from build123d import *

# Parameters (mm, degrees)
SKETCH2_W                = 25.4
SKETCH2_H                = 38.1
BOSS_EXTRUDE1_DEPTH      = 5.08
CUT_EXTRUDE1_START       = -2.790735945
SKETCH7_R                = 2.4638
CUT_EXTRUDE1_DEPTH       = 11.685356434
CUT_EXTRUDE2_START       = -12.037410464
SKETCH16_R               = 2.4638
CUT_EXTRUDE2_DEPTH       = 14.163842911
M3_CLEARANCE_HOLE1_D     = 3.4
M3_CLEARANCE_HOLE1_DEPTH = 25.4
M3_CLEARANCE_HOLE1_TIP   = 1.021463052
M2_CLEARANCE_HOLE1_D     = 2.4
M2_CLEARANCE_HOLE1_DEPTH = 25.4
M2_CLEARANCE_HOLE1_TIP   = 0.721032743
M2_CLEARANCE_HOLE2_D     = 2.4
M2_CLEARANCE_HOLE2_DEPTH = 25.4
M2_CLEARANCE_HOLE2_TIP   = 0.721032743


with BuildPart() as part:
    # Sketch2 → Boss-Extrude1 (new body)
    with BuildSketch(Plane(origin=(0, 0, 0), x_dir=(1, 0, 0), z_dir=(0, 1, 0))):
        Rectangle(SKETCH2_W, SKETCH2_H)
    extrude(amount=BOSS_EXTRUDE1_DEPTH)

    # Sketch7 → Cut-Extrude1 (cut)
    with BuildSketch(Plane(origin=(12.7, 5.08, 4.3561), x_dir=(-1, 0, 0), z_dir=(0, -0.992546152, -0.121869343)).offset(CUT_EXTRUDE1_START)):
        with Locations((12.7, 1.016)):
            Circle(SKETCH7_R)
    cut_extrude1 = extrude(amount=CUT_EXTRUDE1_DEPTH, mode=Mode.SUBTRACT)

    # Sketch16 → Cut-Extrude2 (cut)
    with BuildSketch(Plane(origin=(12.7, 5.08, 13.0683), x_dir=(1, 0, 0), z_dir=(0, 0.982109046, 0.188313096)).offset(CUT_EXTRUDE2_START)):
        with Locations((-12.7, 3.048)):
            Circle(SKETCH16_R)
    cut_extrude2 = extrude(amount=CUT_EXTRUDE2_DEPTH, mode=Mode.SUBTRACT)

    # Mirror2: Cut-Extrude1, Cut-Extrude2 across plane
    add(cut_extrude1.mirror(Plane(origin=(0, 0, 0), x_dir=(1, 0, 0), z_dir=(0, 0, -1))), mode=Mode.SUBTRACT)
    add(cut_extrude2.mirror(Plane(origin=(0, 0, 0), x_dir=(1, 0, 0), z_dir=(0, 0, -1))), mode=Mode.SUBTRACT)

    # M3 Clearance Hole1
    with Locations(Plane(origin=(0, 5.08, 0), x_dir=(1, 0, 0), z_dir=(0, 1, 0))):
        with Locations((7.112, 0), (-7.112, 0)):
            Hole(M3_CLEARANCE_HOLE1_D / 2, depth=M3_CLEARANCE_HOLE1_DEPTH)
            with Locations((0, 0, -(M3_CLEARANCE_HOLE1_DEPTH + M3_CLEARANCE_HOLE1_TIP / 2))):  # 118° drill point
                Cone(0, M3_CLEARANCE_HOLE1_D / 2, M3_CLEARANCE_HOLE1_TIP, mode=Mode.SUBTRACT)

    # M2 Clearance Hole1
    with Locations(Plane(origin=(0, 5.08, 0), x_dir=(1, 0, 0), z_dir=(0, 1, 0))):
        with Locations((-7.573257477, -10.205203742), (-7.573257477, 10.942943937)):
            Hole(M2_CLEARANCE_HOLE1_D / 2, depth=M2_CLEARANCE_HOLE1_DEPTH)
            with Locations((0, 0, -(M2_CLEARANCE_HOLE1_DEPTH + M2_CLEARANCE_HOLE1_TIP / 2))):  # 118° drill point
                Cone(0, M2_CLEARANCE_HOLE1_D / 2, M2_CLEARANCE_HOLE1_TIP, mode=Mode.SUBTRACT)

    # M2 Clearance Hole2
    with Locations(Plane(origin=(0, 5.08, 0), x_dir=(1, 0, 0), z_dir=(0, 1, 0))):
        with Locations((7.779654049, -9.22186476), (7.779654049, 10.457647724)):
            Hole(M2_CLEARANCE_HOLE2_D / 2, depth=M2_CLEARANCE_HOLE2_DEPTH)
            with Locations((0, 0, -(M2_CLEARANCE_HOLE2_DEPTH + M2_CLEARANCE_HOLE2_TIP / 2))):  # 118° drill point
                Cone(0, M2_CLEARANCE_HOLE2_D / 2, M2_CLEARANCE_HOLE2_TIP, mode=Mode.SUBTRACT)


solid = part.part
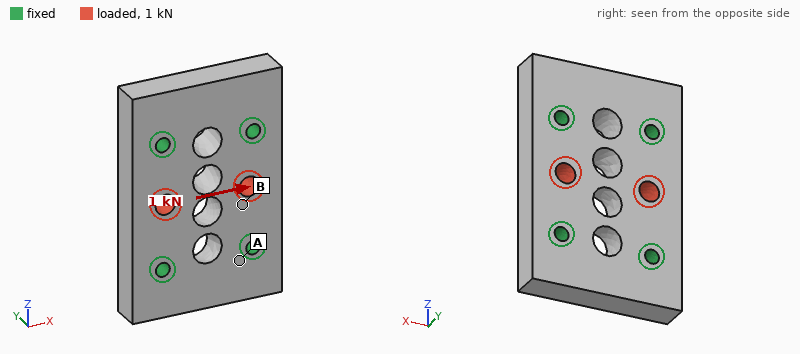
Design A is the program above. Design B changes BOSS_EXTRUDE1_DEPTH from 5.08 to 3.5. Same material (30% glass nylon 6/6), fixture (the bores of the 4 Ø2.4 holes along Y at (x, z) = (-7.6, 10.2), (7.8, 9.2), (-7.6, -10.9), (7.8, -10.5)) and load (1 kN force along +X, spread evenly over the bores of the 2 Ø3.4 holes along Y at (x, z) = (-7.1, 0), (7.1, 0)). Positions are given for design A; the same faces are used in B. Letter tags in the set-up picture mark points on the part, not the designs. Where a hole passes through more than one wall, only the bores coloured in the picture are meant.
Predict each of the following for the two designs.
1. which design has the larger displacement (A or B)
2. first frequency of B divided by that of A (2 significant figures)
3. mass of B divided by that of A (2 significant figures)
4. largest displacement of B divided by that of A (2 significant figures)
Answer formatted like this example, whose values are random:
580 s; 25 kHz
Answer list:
B; 0.78; 0.69; 1.5
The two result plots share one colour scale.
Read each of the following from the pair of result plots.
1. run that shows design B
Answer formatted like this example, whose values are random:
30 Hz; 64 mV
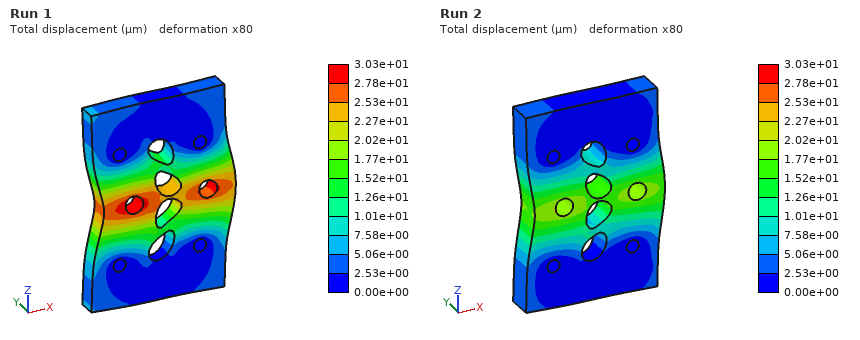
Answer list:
Run 1
